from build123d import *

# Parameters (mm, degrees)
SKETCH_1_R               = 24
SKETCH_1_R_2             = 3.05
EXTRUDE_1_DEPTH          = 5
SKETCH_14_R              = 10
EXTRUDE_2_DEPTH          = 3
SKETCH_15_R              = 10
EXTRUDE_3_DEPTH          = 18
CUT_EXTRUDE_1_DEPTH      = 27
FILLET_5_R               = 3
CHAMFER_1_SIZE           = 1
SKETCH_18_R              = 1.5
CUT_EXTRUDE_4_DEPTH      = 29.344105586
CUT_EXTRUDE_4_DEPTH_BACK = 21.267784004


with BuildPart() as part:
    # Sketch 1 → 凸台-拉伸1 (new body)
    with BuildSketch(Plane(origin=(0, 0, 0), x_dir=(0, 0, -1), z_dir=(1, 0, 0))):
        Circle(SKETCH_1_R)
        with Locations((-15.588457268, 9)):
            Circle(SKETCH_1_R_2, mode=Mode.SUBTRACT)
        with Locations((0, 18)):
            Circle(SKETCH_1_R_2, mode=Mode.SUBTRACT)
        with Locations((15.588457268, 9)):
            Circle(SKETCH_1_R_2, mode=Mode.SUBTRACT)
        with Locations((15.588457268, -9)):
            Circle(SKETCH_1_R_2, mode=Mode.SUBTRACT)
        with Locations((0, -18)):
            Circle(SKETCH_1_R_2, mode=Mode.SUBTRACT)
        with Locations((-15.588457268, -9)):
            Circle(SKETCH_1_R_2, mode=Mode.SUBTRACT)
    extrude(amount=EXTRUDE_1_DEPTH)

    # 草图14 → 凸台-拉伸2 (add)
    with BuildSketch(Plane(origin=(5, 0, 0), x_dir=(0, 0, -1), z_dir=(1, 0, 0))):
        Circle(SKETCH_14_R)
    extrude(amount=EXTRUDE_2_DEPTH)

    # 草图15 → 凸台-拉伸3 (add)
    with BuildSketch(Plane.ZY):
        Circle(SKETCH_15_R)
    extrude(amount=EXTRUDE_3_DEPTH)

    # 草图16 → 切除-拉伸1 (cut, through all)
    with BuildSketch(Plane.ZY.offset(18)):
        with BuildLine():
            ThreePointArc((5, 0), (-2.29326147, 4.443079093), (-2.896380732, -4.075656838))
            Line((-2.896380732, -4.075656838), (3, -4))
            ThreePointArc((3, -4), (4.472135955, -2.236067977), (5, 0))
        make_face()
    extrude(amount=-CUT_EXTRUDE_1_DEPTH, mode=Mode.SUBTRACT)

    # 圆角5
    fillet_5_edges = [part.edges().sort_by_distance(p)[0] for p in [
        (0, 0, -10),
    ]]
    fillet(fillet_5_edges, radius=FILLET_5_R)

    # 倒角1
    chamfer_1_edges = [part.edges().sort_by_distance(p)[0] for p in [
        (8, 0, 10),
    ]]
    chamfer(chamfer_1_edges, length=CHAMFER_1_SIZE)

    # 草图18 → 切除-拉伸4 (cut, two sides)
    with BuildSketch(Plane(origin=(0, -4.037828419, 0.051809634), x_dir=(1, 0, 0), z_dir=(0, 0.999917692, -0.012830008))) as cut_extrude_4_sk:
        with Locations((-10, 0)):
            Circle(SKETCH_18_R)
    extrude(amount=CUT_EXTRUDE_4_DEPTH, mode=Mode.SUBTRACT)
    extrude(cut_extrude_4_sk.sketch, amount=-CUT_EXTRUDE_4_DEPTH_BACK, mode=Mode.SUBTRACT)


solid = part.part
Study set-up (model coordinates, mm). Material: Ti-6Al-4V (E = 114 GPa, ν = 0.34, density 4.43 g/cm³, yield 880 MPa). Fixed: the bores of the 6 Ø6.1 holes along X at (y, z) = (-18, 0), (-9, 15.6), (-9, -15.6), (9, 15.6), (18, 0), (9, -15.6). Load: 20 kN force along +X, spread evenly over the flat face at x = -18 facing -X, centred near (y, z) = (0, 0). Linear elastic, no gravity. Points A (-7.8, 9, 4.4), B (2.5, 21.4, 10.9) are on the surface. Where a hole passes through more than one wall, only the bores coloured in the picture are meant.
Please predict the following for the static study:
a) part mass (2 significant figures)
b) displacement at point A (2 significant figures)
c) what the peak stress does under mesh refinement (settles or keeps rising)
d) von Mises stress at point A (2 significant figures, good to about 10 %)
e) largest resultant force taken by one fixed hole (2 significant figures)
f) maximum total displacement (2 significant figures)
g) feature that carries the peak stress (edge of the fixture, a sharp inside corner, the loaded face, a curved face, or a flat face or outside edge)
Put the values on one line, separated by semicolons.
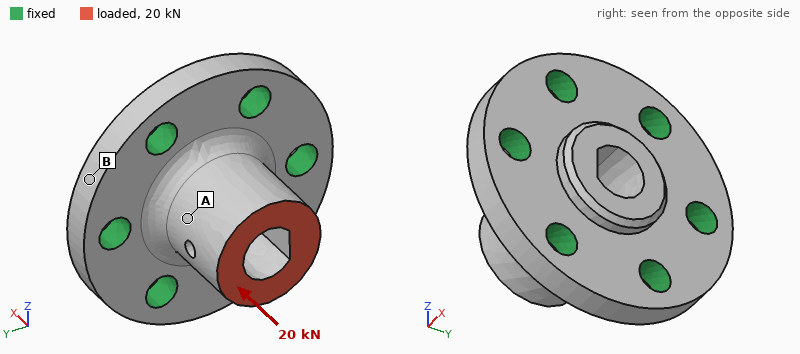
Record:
57 g; 22 µm; keeps rising; 87 MPa; 3.6 kN; 31 µm; edge of the fixture
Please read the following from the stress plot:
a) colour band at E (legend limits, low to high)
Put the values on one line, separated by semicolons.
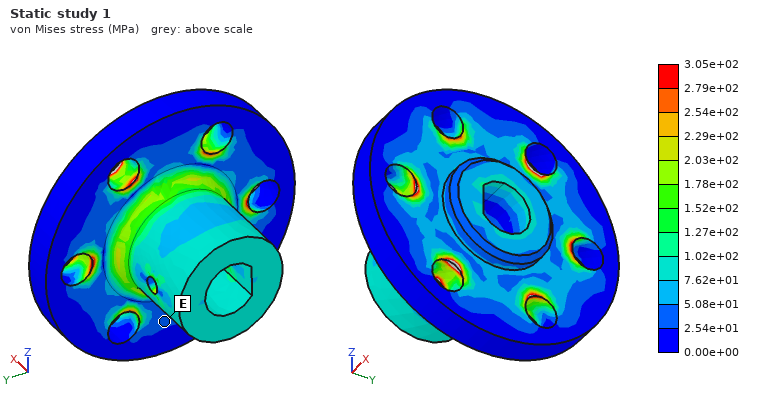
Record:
2.54e+01 to 5.08e+01 MPa
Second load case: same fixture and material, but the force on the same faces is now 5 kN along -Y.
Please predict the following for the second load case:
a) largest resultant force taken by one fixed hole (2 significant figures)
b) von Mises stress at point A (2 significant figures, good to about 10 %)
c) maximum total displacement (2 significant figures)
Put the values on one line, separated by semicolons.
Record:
2.8 kN; 75 MPa; 48 µm
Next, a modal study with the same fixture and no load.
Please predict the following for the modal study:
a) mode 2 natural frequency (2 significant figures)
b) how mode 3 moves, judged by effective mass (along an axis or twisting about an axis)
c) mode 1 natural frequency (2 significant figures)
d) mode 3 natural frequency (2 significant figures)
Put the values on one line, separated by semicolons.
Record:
21 kHz; along X; 21 kHz; 30 kHz
